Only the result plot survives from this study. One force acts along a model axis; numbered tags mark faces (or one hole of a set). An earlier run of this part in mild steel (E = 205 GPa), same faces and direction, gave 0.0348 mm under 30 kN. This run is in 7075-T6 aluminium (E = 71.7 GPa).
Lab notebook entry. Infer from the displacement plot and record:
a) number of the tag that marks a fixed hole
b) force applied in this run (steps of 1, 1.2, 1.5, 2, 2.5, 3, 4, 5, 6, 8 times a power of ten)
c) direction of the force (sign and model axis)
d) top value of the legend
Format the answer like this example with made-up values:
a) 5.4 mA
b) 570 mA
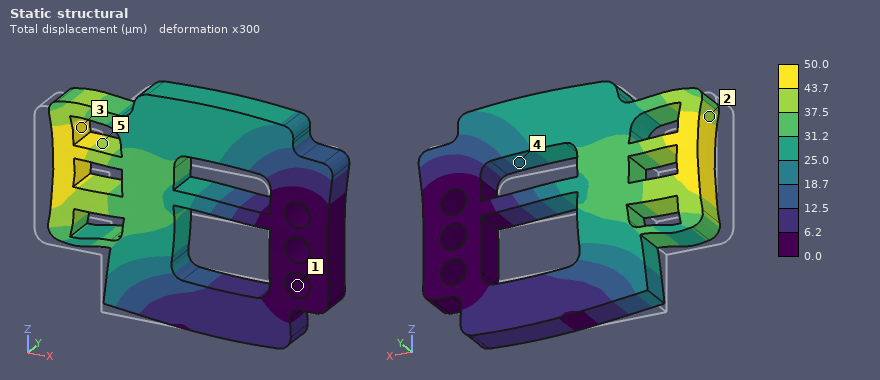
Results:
a) 1
b) 15 kN
c) +X
d) 50.0 µm
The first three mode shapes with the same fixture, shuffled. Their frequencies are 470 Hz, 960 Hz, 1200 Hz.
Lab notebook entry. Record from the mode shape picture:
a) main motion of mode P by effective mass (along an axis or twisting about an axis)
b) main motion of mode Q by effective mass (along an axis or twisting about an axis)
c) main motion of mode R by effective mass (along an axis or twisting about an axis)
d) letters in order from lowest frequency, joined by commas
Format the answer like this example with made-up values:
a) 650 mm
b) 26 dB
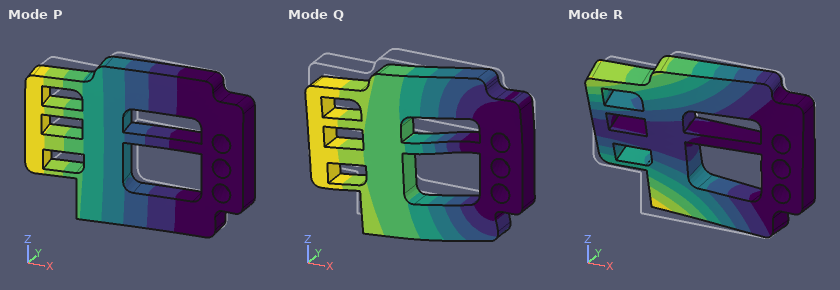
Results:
a) along Y
b) along Z
c) twisting about X
d) P, Q, R
